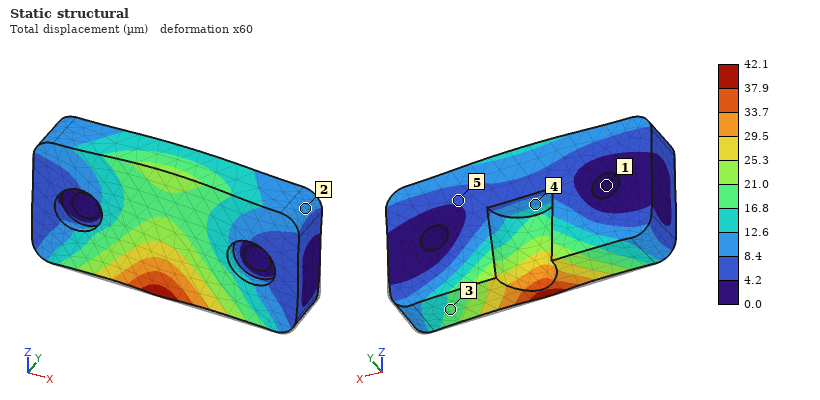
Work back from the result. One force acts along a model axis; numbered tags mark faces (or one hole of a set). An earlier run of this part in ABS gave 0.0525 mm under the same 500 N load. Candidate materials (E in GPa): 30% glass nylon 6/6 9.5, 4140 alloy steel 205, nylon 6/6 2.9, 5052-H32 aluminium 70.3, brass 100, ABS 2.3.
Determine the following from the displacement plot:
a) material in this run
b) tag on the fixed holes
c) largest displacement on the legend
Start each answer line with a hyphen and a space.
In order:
- nylon 6/6
- 1
- 42.1 µm
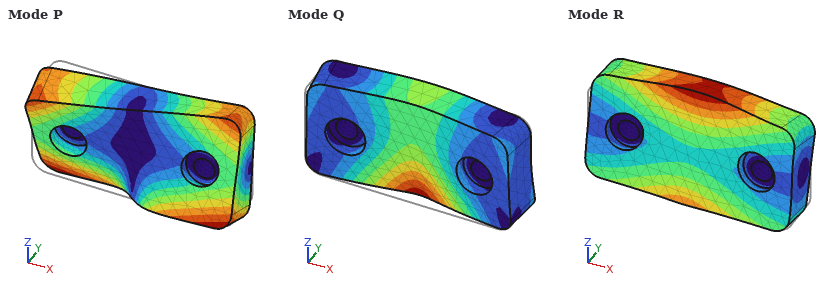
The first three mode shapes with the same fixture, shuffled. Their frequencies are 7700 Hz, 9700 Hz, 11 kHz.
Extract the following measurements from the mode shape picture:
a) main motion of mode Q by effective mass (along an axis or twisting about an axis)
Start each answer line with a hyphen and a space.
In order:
- along Y
